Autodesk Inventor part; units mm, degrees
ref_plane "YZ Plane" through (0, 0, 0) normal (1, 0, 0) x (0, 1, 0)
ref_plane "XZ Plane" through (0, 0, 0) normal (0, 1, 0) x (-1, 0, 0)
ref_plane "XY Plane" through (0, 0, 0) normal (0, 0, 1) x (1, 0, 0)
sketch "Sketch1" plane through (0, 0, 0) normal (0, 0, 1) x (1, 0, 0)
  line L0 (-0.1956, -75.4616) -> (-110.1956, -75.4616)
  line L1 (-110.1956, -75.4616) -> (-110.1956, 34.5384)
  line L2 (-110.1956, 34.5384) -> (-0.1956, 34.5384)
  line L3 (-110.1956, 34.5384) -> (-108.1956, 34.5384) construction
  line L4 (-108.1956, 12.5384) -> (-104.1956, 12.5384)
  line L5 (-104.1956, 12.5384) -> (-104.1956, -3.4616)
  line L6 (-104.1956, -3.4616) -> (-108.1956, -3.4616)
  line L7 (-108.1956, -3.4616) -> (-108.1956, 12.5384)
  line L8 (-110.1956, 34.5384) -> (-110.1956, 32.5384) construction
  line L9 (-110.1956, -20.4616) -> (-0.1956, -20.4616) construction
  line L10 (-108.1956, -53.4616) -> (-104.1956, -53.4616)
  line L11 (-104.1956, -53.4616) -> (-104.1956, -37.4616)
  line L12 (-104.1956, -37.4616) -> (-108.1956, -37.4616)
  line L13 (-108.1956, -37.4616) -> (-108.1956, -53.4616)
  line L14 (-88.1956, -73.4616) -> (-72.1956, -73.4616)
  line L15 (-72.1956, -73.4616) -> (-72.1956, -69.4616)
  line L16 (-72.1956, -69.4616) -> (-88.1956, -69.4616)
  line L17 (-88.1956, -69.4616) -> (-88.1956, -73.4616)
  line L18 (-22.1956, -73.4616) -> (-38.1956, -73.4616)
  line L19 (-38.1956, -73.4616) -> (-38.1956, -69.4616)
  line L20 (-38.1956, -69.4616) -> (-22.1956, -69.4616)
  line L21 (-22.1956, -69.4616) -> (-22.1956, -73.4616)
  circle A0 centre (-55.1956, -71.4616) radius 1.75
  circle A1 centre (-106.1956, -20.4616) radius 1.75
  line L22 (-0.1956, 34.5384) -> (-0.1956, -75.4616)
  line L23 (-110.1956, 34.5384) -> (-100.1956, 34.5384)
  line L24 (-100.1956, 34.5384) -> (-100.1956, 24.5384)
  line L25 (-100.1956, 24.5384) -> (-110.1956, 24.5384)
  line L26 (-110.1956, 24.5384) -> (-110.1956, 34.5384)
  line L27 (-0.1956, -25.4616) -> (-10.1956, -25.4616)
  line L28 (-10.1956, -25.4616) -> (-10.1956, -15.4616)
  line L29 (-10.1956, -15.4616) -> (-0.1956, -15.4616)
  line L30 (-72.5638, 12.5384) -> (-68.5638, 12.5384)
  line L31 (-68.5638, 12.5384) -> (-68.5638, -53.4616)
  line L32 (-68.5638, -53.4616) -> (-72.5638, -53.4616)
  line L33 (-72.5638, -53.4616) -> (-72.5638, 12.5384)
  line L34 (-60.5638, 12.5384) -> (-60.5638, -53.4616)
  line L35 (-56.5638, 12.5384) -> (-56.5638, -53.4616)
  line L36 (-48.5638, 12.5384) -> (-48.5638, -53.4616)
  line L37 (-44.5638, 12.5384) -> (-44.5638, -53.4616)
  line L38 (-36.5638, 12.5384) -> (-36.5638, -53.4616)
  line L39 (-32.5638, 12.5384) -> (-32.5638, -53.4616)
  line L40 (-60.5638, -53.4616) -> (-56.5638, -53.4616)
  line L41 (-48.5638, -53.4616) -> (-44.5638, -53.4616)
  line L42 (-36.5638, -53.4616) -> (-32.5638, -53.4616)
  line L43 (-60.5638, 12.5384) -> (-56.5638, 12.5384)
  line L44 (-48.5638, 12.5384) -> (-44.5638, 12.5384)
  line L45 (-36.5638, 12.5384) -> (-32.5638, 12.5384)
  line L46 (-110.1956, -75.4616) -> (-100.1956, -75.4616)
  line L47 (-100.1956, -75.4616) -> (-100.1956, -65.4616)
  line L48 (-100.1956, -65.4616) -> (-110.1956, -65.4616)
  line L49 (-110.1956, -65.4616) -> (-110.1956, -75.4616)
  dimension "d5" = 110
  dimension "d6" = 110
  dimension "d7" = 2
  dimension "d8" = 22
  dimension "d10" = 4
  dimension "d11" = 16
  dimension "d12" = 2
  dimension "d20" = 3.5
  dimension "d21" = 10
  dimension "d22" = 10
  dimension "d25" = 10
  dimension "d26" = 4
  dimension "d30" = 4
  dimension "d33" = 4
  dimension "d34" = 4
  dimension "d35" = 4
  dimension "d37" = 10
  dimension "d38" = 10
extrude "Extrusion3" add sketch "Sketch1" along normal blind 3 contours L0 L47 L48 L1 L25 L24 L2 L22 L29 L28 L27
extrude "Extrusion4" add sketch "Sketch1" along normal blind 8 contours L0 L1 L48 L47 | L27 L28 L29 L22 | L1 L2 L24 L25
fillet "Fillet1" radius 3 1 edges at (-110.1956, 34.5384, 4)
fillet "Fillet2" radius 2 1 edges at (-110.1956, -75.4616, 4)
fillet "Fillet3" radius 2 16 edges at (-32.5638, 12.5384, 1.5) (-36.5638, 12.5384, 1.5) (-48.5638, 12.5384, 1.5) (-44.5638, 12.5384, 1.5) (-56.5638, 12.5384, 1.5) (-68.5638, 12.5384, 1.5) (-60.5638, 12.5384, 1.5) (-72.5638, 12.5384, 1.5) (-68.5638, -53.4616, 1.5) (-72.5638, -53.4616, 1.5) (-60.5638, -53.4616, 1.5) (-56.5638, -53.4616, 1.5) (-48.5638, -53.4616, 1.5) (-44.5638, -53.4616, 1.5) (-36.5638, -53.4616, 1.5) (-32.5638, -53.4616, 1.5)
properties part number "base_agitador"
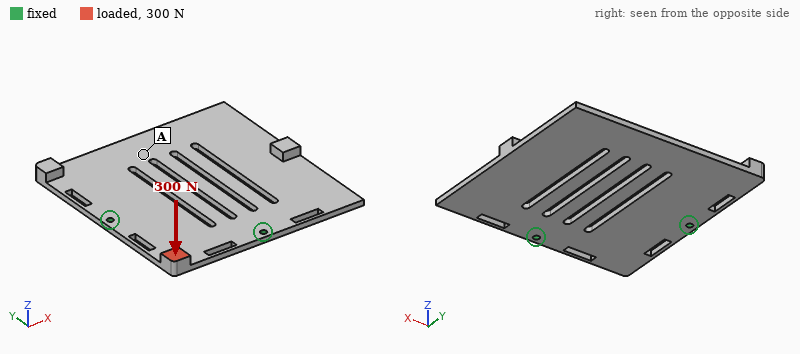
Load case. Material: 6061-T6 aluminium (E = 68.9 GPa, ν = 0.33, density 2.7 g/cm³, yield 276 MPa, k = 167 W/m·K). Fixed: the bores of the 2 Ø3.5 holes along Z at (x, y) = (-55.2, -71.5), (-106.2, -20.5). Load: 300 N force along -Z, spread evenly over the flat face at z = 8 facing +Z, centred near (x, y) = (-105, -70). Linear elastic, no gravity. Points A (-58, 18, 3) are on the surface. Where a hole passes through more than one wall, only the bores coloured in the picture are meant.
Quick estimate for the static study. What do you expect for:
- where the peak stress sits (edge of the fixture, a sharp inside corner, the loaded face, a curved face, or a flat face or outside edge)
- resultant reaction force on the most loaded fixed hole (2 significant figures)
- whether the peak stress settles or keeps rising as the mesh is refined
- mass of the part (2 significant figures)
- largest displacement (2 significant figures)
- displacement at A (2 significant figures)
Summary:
edge of the fixture
150 N
keeps rising
91 g
1.6 mm
0.50 mm
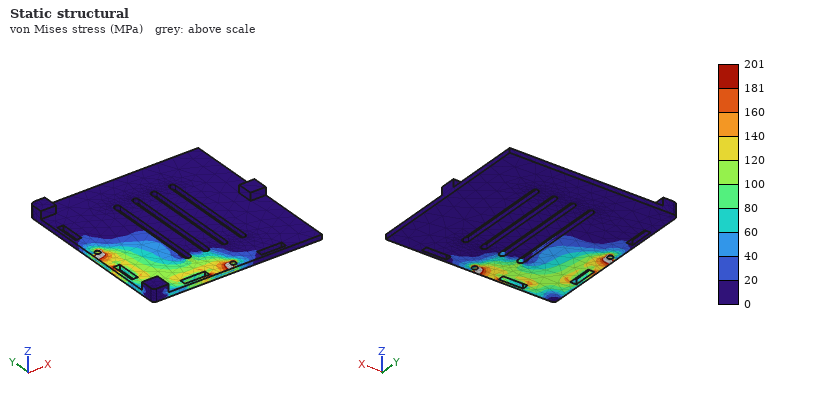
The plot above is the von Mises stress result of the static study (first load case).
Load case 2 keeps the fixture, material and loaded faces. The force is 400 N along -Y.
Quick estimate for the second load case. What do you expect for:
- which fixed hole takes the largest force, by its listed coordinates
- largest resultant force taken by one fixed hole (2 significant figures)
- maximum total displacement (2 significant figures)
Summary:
(-106.2, -20.5)
340 N
0.38 mm
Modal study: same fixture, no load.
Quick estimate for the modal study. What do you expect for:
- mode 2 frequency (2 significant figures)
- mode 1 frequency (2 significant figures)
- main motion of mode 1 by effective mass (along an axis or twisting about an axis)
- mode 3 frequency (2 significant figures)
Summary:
540 Hz
220 Hz
along Z
950 Hz
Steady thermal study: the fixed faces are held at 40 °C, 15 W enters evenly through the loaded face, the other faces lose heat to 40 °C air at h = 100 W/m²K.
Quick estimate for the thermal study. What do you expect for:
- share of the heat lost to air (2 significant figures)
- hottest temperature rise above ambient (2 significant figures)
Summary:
54 %
38 K
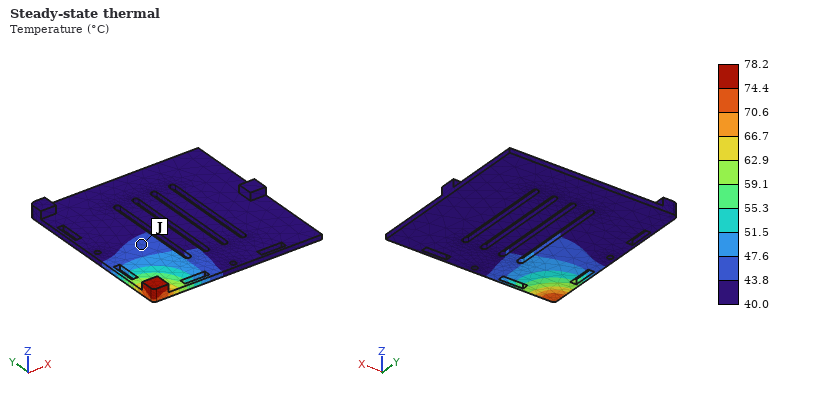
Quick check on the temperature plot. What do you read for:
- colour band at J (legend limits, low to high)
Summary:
43.8 to 47.6 °C
